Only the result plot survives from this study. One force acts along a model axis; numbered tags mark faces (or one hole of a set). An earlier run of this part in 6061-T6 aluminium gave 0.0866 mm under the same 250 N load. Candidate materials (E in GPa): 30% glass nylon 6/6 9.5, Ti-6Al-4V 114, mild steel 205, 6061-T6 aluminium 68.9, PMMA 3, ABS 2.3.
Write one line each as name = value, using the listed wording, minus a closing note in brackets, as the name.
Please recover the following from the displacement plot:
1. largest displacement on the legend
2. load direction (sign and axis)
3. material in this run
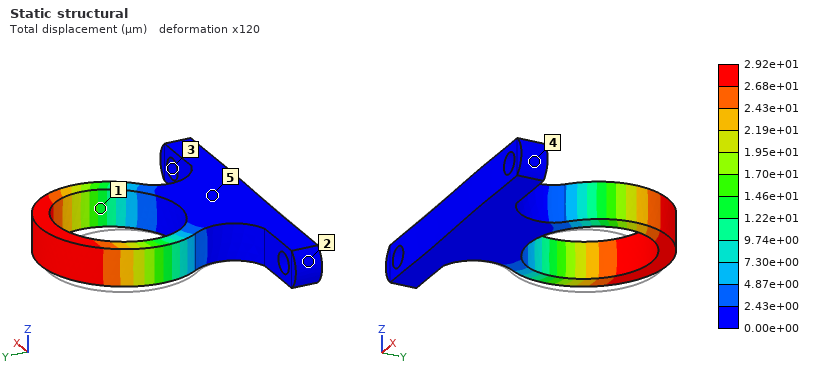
largest displacement on the legend = 2.92e+01 µm
load direction = +X
material in this run = mild steel
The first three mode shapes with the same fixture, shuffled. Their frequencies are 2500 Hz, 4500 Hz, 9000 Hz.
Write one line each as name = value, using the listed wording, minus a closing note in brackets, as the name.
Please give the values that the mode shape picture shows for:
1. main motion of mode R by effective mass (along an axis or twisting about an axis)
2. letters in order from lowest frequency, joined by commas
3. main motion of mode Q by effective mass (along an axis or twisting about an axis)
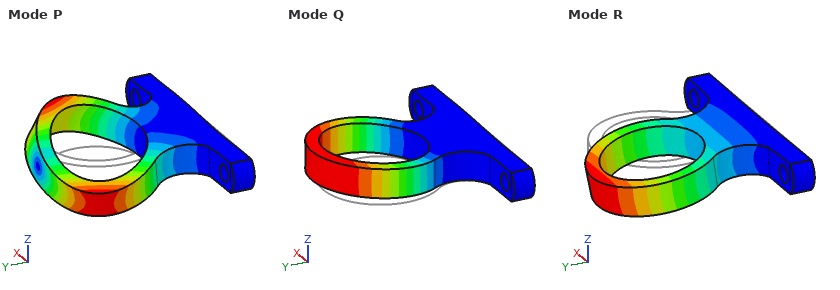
main motion of mode R by effective mass = along Z
letters in order from lowest frequency, joined by commas = R, Q, P
main motion of mode Q by effective mass = along X
